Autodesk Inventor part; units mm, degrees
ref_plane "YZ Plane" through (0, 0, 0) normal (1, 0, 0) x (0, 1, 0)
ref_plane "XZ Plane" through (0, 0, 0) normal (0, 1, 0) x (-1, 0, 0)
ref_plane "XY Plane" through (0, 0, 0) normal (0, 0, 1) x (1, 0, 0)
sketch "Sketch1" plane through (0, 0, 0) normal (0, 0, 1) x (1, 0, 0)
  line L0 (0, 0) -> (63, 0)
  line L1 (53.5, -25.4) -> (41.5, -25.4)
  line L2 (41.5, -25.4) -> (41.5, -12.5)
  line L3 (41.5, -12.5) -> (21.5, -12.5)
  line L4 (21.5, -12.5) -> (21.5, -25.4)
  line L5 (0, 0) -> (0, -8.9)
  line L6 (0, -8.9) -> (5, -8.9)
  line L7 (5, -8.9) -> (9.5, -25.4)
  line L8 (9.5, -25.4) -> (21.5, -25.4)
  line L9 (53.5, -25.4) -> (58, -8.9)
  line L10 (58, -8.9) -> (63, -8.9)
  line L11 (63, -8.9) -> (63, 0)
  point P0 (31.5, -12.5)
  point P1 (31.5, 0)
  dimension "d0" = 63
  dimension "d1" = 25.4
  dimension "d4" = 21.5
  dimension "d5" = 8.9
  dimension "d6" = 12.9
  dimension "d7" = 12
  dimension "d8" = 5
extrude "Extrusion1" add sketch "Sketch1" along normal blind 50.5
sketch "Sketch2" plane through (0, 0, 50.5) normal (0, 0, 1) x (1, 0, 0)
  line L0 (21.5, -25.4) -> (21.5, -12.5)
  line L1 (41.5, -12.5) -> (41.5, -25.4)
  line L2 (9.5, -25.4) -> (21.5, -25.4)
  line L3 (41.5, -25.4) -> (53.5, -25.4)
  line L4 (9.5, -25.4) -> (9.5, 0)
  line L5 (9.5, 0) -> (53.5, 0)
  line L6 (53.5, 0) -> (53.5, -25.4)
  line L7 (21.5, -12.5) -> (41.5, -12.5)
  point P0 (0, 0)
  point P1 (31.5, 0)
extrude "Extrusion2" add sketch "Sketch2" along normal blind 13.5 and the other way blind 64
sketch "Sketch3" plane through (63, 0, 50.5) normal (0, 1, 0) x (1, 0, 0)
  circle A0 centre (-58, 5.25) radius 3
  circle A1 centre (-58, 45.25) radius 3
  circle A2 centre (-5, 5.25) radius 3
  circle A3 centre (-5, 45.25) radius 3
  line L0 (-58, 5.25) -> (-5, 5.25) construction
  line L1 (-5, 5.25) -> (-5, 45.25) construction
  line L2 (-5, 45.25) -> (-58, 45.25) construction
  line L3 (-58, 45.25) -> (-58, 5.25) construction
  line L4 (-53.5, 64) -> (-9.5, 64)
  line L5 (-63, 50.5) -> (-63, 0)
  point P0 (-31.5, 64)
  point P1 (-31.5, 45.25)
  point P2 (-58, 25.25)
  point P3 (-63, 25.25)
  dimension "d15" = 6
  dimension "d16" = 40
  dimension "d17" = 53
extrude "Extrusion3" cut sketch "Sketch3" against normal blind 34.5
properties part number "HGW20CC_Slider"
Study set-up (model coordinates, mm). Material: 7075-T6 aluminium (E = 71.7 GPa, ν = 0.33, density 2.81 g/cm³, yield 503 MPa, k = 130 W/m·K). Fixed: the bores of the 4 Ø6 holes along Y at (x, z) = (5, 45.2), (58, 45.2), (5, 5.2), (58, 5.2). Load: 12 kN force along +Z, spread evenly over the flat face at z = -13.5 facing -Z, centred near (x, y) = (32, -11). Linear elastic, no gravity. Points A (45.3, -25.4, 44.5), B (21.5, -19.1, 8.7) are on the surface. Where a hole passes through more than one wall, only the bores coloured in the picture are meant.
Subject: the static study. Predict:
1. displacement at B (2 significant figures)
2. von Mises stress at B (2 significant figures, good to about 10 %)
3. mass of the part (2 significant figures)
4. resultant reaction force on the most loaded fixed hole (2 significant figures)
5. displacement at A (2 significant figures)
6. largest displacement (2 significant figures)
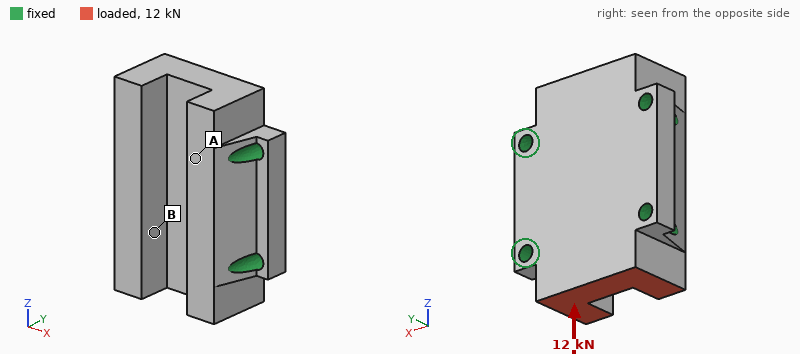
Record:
4.6 µm
13 MPa
220 g
4.0 kN
1.7 µm
9.7 µm
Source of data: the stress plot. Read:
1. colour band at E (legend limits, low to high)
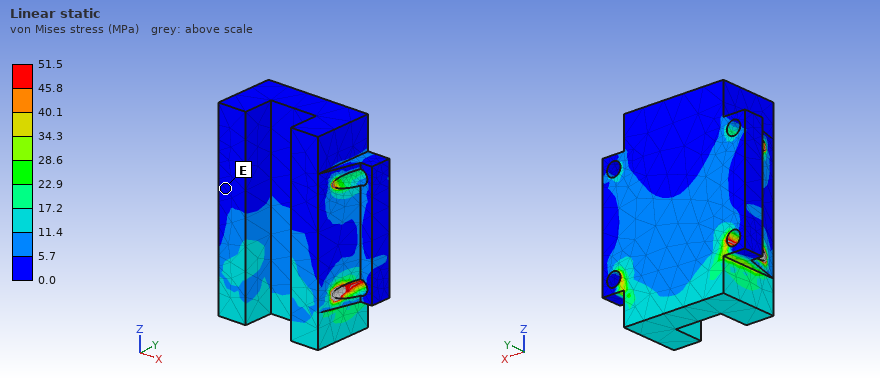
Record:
0.0 to 5.7 MPa
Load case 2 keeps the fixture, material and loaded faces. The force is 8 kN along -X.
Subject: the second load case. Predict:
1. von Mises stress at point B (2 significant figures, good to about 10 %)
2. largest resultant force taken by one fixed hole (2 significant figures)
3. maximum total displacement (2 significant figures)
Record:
17 MPa
4.9 kN
23 µm
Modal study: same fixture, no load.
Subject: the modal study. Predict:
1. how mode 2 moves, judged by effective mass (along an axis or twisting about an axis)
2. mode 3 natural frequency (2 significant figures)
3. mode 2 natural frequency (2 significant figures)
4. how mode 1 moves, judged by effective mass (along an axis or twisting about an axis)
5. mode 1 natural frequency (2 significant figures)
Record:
twisting about X
20 kHz
15 kHz
along Y
14 kHz
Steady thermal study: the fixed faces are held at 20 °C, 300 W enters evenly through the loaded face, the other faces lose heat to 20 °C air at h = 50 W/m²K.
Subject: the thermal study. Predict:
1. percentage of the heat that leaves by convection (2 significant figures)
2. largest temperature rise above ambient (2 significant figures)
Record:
3.8 %
74 K
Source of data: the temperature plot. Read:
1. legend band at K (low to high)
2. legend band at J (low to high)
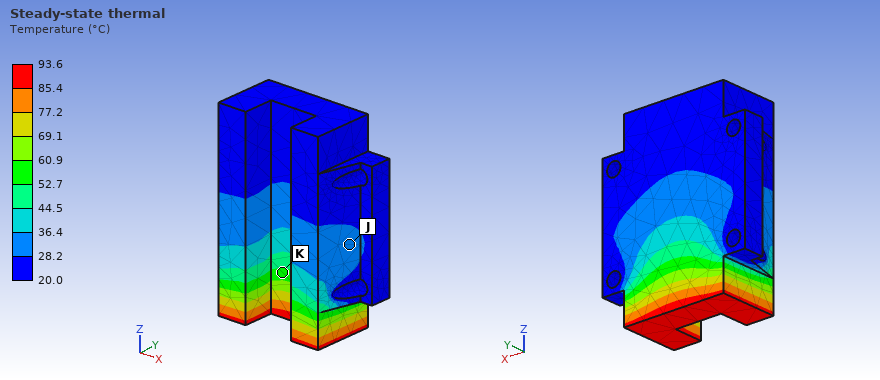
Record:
52.7 to 60.9 °C
28.2 to 36.4 °C
